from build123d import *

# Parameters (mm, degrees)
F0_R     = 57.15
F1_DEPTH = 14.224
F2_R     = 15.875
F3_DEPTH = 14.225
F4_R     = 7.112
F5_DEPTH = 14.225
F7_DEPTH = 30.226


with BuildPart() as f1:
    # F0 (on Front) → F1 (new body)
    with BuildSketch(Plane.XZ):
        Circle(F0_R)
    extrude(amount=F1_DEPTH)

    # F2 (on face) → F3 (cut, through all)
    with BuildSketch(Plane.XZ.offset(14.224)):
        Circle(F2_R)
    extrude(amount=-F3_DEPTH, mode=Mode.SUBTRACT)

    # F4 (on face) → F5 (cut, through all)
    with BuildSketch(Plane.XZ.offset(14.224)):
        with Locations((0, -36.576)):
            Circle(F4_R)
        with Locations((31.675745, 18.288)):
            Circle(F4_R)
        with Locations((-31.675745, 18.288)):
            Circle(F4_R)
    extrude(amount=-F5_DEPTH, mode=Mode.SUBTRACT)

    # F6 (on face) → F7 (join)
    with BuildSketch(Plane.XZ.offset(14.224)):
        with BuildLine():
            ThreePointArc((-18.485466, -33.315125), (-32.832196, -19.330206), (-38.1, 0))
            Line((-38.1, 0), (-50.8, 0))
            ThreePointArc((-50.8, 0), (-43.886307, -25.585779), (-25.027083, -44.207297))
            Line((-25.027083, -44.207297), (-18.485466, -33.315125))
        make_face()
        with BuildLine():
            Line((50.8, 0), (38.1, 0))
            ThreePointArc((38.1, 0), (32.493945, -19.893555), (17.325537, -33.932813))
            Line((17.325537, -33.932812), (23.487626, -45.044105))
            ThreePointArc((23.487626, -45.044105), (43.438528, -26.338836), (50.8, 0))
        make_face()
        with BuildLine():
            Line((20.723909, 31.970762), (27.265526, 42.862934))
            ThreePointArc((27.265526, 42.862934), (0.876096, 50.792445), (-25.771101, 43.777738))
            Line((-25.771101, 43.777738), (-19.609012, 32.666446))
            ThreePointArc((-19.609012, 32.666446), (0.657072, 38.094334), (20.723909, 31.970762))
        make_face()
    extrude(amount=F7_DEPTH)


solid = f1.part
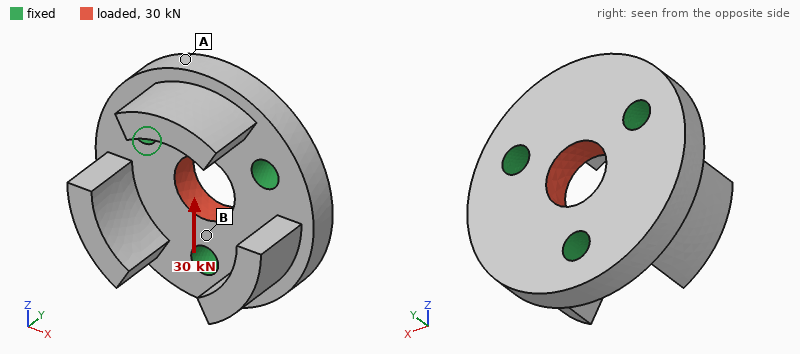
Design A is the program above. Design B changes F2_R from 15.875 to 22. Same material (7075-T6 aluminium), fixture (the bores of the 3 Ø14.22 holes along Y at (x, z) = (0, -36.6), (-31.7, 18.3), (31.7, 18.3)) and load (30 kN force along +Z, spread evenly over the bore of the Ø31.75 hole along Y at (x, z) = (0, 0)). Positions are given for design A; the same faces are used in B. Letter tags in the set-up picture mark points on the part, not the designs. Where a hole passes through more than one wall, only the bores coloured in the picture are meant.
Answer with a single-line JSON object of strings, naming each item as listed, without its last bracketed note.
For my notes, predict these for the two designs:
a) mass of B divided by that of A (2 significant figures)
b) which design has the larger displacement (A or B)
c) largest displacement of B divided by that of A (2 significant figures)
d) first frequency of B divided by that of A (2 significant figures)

{"mass of B divided by that of A": "0.94", "which design has the larger displacement": "A", "largest displacement of B divided by that of A": "0.83", "first frequency of B divided by that of A": "0.96"}
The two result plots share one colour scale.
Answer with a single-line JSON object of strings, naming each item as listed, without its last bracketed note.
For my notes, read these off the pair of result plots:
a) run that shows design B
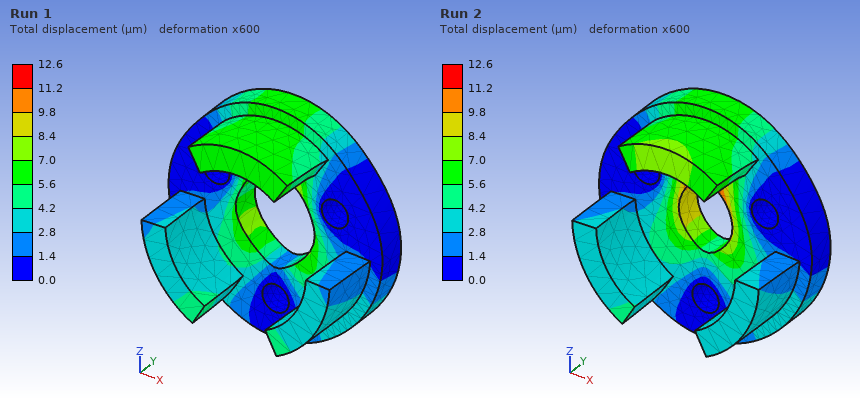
{"run that shows design B": "Run 1"}
